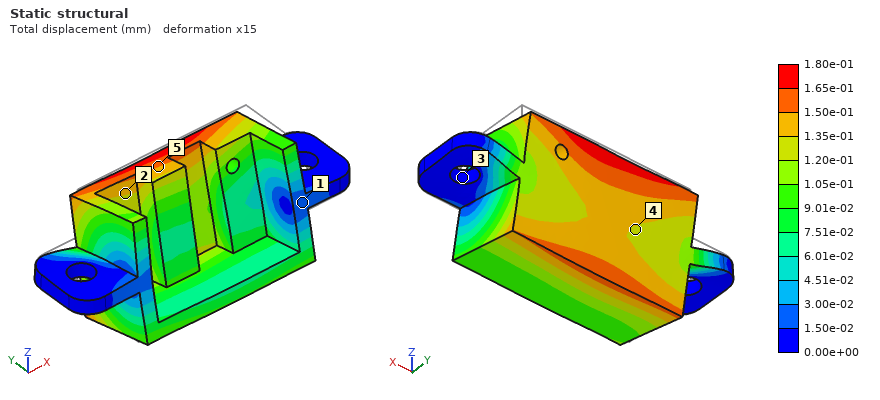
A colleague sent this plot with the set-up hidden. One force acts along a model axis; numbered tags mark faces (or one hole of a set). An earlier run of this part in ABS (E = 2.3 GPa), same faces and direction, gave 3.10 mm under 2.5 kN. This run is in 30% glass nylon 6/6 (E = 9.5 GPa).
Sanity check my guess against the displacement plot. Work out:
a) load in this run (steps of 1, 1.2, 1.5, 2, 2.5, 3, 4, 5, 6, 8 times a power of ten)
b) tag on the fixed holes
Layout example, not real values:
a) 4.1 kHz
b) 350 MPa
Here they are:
a) 600 N
b) 3
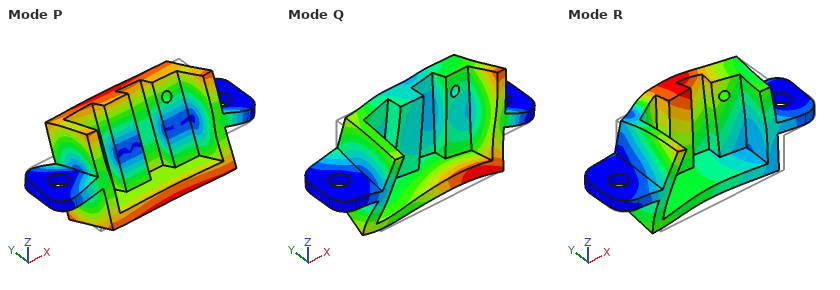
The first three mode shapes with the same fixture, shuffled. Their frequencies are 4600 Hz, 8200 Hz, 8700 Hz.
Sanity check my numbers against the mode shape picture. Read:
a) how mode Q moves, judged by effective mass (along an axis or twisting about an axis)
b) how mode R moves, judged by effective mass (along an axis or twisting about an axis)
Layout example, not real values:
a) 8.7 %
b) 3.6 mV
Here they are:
a) along Z
b) along Y
